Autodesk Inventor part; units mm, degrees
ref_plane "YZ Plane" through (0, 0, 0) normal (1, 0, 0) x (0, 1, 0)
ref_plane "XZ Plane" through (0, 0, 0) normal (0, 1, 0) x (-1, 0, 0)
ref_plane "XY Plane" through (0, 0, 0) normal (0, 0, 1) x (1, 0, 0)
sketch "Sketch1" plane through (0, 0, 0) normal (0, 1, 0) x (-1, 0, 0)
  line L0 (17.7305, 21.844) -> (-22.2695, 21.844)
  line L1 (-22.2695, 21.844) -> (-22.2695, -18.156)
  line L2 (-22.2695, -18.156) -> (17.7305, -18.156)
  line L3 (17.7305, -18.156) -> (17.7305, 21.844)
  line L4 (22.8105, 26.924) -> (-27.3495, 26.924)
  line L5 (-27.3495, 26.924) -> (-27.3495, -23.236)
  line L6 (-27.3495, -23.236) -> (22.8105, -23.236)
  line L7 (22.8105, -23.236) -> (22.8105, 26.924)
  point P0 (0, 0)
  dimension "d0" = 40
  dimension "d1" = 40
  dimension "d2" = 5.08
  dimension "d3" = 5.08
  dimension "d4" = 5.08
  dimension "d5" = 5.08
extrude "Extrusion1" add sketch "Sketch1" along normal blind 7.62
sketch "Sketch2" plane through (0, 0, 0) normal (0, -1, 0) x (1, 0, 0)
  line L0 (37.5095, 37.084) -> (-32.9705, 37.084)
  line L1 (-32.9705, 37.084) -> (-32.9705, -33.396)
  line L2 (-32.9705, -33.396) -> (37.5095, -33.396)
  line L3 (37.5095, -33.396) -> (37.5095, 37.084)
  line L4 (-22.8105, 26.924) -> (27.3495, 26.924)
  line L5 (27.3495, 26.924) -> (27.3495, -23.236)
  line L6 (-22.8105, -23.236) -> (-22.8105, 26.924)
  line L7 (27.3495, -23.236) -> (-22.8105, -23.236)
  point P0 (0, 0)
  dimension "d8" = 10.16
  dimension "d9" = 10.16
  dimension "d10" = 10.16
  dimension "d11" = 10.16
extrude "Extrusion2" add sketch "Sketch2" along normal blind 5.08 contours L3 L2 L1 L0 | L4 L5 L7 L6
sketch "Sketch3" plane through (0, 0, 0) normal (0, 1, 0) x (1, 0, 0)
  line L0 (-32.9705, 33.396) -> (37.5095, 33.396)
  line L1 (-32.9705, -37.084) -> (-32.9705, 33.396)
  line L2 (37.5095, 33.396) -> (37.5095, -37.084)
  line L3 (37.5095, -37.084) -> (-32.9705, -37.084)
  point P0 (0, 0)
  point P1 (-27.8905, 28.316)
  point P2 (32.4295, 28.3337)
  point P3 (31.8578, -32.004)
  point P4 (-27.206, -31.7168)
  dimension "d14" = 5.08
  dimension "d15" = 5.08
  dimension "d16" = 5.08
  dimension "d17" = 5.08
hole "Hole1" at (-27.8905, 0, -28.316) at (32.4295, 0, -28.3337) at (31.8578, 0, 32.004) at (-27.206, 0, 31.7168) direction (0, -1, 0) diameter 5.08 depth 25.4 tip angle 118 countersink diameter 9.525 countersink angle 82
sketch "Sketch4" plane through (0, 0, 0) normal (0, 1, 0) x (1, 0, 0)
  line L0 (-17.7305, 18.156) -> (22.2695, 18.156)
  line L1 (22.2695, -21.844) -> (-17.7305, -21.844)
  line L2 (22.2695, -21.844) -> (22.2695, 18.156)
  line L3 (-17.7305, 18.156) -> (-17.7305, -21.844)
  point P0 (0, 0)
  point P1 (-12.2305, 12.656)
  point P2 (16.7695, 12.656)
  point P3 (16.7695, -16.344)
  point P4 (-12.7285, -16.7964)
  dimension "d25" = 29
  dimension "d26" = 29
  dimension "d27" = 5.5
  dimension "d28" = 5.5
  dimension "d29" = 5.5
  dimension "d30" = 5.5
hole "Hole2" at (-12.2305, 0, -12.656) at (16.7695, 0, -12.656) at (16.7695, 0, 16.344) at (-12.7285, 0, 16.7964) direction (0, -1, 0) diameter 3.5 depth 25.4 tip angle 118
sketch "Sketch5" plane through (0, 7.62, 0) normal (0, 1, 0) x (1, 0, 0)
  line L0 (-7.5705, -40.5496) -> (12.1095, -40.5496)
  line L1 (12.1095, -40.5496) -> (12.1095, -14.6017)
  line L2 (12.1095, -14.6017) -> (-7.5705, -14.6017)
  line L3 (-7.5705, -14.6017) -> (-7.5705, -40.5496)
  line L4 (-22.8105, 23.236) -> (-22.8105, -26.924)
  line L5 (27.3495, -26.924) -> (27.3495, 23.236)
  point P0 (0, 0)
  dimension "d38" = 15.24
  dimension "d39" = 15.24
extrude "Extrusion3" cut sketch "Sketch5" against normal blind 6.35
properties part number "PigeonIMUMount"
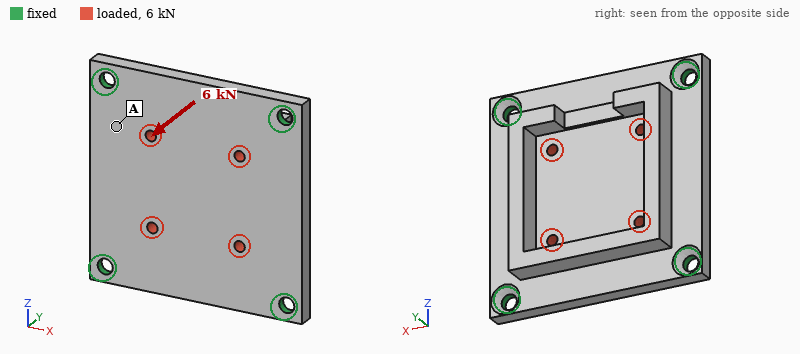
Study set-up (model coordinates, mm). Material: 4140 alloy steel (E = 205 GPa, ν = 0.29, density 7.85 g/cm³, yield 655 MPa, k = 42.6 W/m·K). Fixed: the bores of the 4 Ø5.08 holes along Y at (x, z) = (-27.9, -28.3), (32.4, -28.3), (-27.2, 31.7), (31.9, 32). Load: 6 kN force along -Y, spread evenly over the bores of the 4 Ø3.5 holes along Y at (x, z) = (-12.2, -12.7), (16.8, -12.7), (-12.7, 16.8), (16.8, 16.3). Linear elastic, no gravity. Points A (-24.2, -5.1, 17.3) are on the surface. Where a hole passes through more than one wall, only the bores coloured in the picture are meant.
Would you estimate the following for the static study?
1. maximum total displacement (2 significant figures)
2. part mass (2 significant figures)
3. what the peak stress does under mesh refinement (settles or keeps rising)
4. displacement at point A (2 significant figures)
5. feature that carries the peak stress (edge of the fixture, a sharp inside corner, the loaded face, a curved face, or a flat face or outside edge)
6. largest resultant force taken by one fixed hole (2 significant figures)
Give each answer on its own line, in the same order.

46 µm
240 g
keeps rising
16 µm
edge of the fixture
2.5 kN
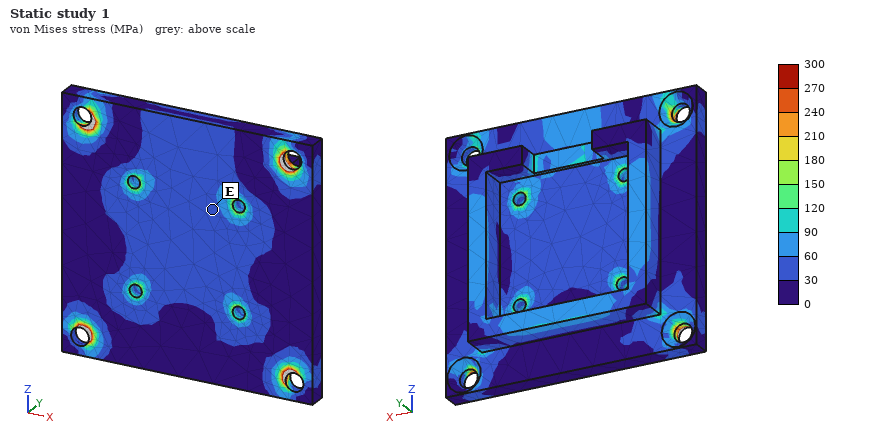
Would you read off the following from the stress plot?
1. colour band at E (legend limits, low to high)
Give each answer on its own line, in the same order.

30 to 60 MPa
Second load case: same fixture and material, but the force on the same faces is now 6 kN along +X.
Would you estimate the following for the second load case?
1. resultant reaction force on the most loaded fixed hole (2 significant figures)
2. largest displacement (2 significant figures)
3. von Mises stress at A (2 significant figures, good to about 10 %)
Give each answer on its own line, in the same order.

1.6 kN
3.7 µm
13 MPa
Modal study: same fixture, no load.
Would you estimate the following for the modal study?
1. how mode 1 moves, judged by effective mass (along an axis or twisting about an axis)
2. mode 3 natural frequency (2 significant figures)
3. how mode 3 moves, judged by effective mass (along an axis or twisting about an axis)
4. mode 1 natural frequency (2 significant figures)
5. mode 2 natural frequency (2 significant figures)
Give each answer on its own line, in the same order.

along Y
8800 Hz
twisting about Z
5200 Hz
8000 Hz
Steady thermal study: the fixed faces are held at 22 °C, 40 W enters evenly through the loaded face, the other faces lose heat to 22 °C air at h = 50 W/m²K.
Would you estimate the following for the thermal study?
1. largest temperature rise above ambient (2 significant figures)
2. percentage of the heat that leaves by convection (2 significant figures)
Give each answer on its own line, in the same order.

39 K
36 %
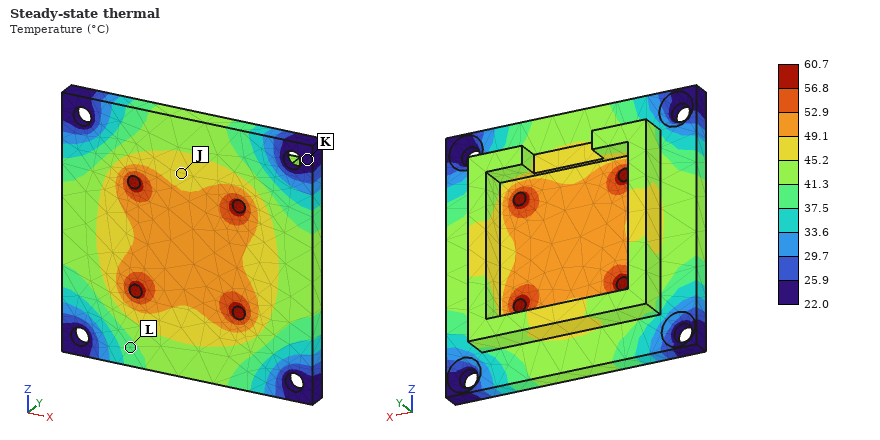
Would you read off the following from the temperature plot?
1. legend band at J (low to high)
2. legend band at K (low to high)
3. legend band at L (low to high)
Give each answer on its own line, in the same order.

45.2 to 49.1 °C
22.0 to 25.9 °C
37.5 to 41.3 °C
